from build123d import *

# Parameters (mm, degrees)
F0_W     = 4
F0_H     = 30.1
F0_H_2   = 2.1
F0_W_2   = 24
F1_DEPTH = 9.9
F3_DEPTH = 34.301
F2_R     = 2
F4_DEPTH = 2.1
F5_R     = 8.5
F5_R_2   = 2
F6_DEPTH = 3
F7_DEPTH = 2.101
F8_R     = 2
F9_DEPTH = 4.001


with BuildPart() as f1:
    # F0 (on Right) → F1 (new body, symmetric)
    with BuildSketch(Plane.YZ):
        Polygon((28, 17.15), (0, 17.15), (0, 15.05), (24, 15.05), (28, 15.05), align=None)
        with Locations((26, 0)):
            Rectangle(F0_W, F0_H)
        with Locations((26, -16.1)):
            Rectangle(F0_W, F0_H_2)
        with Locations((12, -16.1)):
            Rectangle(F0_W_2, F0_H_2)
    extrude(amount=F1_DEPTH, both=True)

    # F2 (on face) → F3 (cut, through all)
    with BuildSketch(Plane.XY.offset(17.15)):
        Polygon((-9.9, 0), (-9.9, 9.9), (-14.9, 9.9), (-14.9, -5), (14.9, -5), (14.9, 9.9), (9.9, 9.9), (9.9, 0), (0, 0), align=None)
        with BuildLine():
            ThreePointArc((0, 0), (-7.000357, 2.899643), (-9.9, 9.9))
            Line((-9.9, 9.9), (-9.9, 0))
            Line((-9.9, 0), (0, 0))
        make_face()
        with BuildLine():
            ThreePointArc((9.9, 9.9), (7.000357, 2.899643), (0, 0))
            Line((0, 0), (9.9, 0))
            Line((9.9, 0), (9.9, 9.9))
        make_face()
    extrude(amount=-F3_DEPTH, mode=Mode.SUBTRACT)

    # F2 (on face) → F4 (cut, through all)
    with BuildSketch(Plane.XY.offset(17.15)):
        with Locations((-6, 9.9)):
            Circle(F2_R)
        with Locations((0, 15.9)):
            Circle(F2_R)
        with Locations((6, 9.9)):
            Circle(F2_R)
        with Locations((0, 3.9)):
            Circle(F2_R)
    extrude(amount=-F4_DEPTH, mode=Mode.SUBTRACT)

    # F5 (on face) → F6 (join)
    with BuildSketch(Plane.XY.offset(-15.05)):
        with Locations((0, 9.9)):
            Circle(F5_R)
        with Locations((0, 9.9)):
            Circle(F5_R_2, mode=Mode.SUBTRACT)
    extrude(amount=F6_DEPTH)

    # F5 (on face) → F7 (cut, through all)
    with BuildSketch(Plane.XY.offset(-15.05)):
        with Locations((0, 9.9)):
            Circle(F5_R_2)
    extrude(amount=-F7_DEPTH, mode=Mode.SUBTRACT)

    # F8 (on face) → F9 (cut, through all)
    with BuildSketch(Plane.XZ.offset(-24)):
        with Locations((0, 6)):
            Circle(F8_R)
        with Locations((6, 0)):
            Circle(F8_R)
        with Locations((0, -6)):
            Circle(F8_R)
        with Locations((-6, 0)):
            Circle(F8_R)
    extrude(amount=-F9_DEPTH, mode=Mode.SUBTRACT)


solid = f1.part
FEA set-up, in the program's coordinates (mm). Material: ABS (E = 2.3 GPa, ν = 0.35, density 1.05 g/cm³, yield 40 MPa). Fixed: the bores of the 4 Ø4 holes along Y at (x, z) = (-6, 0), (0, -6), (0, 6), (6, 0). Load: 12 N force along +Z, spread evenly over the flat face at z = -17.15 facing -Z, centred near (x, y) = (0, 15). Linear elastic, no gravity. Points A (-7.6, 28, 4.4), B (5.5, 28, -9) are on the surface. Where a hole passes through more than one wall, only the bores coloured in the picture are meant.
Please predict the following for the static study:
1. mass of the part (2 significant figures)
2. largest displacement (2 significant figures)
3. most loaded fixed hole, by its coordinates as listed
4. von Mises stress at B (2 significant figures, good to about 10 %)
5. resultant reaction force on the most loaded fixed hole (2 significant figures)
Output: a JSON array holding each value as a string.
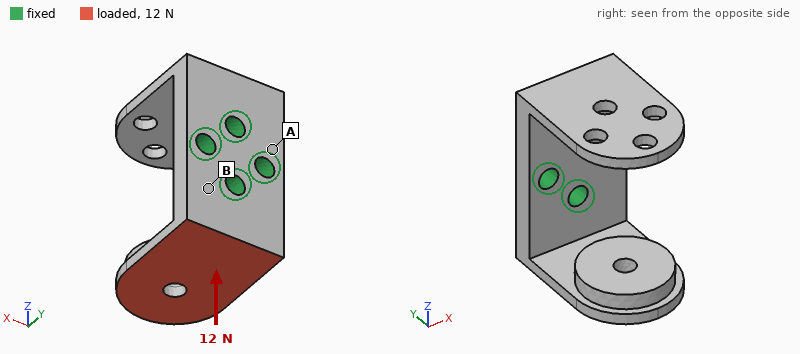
["5.1 g", "0.51 mm", "(0, -6)", "1.7 MPa", "11 N"]
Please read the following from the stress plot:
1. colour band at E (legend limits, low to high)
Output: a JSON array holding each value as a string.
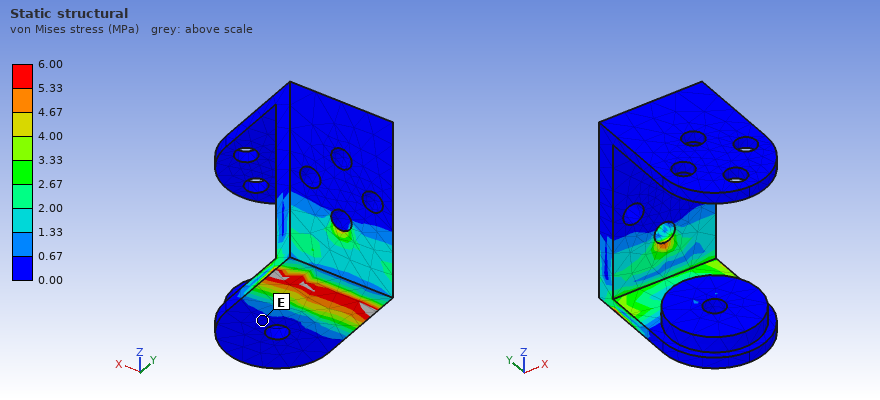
["0.00 to 0.67 MPa"]
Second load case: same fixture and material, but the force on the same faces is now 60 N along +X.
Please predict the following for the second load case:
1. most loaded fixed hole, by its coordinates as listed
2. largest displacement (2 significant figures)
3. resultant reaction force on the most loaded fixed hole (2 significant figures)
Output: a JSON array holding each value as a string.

["(0, -6)", "0.47 mm", "67 N"]
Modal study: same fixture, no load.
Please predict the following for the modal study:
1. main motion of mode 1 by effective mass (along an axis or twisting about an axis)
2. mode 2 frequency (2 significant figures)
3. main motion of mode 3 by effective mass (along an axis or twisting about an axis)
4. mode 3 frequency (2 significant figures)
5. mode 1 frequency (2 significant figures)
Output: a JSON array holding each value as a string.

["along Z", "910 Hz", "along X", "1400 Hz", "660 Hz"]
